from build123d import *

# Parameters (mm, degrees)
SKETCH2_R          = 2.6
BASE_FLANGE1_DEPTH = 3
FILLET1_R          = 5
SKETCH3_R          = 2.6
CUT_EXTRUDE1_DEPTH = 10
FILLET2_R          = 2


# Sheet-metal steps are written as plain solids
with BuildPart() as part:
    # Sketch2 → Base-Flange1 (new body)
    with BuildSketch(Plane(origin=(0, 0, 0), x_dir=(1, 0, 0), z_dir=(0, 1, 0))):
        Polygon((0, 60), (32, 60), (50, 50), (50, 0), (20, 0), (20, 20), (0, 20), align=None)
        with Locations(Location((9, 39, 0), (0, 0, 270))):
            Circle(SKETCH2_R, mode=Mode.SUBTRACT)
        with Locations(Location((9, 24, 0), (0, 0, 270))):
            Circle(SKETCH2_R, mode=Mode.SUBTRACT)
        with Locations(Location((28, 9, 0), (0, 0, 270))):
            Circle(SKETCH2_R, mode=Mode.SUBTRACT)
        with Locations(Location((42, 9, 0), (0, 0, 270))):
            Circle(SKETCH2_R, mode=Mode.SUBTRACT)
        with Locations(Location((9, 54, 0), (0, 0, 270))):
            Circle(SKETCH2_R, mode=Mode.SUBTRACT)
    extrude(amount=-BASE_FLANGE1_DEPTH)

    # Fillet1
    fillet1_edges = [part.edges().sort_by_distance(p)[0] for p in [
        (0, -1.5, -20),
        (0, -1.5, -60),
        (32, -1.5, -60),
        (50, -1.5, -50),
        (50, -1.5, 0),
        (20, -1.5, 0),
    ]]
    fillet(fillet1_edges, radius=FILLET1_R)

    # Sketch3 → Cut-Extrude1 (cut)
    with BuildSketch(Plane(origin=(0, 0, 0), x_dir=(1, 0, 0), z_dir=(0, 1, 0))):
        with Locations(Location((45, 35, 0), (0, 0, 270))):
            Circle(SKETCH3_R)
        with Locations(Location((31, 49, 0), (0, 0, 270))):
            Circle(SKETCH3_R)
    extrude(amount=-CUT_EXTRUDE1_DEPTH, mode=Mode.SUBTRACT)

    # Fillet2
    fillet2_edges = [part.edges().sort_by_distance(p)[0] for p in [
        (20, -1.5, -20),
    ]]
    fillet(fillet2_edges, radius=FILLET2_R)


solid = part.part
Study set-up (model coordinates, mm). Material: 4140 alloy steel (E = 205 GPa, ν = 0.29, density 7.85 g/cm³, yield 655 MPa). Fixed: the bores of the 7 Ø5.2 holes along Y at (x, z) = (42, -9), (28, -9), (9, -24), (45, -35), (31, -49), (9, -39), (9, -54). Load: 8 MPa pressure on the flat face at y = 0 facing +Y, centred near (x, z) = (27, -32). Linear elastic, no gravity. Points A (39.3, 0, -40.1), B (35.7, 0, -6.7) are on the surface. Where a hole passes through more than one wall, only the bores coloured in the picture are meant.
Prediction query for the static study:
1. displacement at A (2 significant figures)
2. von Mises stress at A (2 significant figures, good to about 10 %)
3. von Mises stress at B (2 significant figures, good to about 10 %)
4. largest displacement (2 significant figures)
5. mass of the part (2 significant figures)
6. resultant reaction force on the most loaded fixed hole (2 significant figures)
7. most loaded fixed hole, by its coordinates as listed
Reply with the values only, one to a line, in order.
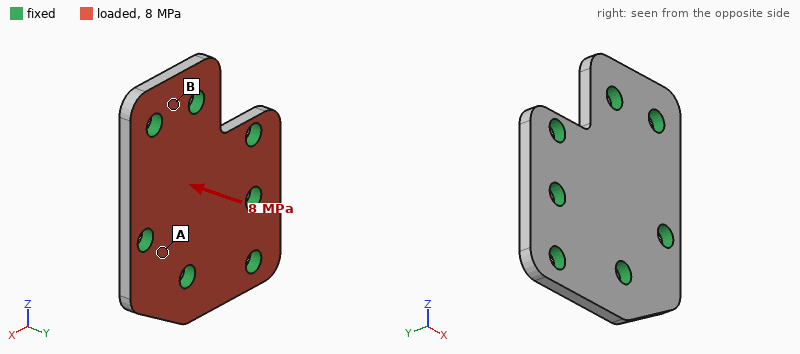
6.8 µm
170 MPa
77 MPa
39 µm
55 g
3.7 kN
(31, -49)
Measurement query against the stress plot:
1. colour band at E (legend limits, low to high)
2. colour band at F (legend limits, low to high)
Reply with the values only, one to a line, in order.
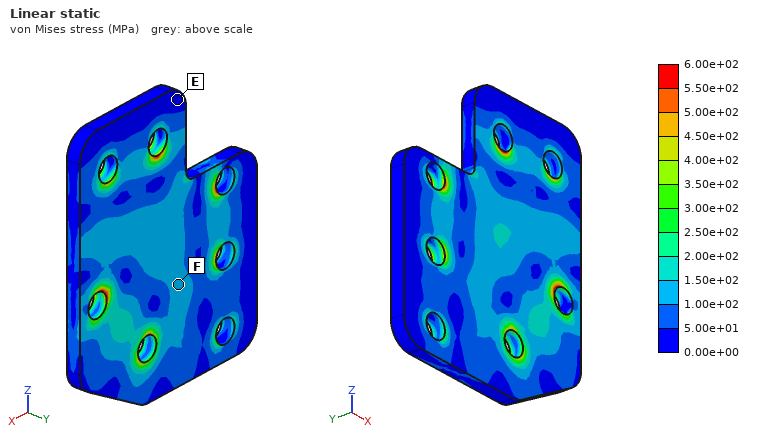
0.00e+00 to 5.00e+01 MPa
1.00e+02 to 1.50e+02 MPa
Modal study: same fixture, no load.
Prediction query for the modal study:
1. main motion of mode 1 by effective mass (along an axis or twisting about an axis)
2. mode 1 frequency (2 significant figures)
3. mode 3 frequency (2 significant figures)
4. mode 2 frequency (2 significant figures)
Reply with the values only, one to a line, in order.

along Y
18 kHz
27 kHz
20 kHz
